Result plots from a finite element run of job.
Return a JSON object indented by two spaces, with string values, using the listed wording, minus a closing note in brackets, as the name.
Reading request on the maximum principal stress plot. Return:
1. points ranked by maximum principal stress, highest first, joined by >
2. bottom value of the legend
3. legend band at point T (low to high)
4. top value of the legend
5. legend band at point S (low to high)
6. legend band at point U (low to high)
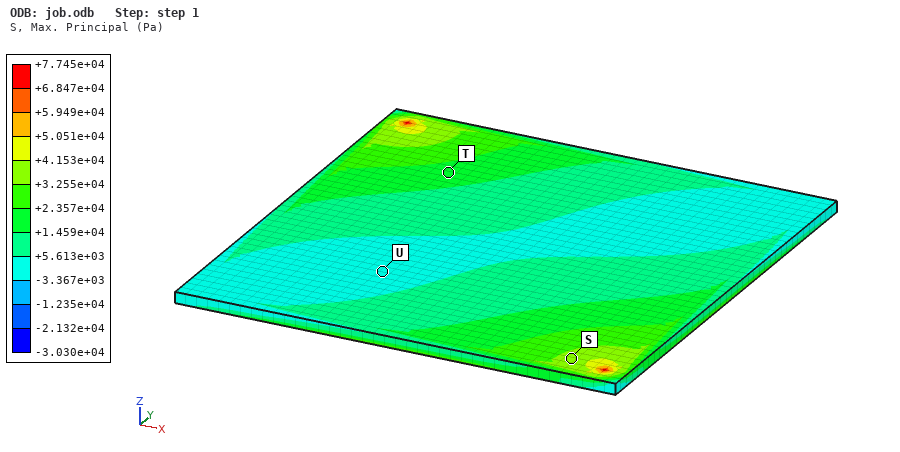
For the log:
{
  "points ranked by maximum principal stress, highest first, joined by >": "S > T > U",
  "bottom value of the legend": "-3.030e+04 Pa",
  "legend band at point T": "+1.459e+04 to +2.357e+04 Pa",
  "top value of the legend": "+7.745e+04 Pa",
  "legend band at point S": "+3.255e+04 to +4.153e+04 Pa",
  "legend band at point U": "-3.367e+03 to +5.613e+03 Pa"
}
